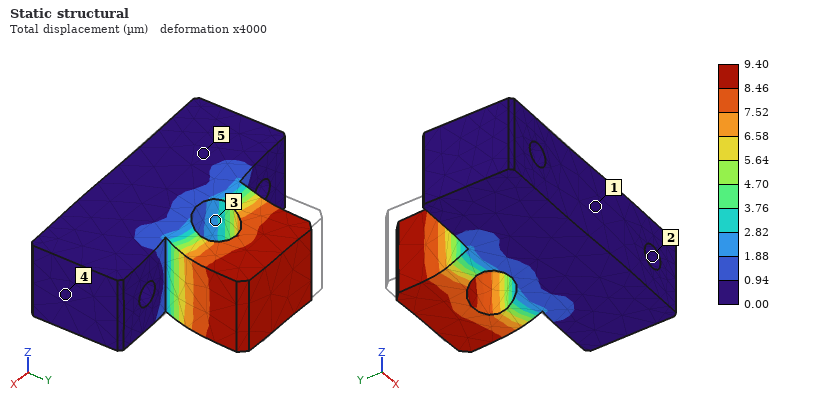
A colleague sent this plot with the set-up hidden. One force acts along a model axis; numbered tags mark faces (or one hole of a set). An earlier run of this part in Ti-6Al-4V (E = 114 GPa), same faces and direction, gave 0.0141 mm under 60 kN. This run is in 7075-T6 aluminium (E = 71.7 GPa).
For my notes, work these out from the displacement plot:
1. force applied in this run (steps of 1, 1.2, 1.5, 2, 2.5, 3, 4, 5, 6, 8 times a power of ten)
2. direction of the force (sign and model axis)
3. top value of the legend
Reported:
25 kN
+X
9.40 µm
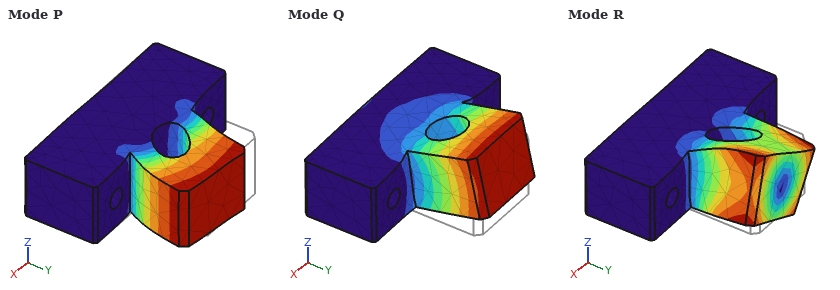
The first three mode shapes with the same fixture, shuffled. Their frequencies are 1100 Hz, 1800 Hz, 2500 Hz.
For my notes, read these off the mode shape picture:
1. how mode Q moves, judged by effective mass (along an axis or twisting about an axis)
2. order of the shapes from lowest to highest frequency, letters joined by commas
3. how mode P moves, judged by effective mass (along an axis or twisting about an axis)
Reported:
along Z
Q, P, R
along X
